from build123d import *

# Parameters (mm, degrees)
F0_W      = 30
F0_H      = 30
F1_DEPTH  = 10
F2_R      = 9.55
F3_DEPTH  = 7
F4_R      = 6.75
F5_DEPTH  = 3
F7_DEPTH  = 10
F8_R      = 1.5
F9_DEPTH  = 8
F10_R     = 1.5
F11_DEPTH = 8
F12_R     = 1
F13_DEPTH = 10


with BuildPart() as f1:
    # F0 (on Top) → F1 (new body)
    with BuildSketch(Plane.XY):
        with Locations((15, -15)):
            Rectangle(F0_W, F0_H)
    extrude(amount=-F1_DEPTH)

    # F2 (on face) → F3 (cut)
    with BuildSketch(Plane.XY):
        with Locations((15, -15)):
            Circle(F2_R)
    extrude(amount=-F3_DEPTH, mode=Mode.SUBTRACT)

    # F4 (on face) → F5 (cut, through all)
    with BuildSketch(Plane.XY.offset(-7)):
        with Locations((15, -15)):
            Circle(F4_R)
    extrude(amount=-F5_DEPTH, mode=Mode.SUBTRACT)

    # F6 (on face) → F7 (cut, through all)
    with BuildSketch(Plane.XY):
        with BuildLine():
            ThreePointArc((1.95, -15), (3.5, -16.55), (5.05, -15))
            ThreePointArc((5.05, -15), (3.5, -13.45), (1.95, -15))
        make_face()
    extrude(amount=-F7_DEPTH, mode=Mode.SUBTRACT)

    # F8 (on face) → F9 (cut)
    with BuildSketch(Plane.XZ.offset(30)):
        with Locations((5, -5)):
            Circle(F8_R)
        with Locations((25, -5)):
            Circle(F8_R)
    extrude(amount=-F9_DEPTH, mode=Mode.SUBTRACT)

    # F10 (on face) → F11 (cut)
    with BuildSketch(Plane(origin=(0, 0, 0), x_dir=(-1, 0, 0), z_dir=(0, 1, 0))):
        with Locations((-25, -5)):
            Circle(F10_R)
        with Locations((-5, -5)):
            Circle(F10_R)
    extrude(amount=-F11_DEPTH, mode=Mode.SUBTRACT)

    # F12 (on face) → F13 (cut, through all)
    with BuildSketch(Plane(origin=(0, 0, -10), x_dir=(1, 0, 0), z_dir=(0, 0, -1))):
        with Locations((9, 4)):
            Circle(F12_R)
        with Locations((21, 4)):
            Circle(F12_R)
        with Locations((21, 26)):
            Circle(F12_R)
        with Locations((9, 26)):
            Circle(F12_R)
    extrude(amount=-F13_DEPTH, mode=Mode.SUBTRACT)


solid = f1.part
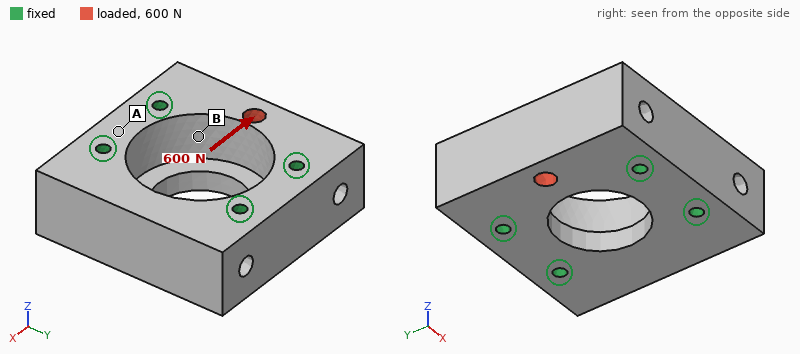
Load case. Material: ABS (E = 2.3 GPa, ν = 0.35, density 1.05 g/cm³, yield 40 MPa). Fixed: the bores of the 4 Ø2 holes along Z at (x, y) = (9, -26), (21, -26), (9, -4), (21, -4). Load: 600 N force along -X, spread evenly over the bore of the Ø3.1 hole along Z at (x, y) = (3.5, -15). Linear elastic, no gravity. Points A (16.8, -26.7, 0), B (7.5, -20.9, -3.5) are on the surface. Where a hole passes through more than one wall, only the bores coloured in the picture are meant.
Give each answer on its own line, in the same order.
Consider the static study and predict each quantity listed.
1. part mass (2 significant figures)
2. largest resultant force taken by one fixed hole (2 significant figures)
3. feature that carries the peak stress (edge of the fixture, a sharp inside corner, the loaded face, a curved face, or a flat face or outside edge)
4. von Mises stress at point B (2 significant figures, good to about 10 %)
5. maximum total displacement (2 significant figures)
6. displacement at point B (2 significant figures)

6.4 g
350 N
a curved face
14 MPa
0.13 mm
0.035 mm
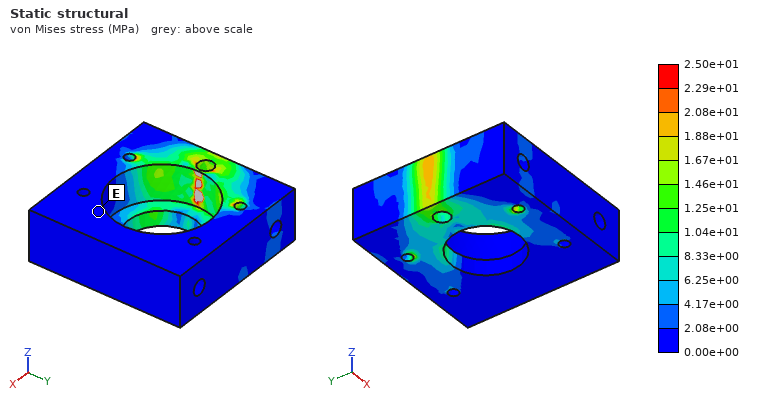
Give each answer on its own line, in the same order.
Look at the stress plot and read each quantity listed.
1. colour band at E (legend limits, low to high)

0.00e+00 to 2.08e+00 MPa
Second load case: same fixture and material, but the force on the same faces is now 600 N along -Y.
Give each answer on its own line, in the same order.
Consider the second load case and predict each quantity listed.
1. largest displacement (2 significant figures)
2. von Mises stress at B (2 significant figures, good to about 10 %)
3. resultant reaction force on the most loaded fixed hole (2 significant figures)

56 µm
8.2 MPa
330 N
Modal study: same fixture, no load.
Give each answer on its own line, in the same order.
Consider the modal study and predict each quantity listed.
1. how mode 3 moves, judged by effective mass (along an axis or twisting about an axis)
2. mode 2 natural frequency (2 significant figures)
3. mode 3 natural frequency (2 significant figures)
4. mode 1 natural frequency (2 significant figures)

along Y
11 kHz
14 kHz
11 kHz
